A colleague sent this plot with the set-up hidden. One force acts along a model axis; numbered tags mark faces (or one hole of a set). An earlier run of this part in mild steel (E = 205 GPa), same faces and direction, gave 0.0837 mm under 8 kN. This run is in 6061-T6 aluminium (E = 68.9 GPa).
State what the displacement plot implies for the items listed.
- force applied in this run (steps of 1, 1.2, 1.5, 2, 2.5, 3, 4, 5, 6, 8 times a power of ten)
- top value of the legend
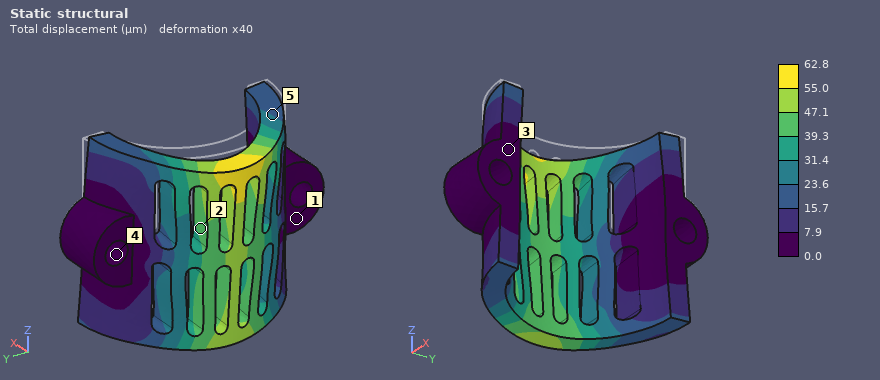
2 kN
62.8 µm
